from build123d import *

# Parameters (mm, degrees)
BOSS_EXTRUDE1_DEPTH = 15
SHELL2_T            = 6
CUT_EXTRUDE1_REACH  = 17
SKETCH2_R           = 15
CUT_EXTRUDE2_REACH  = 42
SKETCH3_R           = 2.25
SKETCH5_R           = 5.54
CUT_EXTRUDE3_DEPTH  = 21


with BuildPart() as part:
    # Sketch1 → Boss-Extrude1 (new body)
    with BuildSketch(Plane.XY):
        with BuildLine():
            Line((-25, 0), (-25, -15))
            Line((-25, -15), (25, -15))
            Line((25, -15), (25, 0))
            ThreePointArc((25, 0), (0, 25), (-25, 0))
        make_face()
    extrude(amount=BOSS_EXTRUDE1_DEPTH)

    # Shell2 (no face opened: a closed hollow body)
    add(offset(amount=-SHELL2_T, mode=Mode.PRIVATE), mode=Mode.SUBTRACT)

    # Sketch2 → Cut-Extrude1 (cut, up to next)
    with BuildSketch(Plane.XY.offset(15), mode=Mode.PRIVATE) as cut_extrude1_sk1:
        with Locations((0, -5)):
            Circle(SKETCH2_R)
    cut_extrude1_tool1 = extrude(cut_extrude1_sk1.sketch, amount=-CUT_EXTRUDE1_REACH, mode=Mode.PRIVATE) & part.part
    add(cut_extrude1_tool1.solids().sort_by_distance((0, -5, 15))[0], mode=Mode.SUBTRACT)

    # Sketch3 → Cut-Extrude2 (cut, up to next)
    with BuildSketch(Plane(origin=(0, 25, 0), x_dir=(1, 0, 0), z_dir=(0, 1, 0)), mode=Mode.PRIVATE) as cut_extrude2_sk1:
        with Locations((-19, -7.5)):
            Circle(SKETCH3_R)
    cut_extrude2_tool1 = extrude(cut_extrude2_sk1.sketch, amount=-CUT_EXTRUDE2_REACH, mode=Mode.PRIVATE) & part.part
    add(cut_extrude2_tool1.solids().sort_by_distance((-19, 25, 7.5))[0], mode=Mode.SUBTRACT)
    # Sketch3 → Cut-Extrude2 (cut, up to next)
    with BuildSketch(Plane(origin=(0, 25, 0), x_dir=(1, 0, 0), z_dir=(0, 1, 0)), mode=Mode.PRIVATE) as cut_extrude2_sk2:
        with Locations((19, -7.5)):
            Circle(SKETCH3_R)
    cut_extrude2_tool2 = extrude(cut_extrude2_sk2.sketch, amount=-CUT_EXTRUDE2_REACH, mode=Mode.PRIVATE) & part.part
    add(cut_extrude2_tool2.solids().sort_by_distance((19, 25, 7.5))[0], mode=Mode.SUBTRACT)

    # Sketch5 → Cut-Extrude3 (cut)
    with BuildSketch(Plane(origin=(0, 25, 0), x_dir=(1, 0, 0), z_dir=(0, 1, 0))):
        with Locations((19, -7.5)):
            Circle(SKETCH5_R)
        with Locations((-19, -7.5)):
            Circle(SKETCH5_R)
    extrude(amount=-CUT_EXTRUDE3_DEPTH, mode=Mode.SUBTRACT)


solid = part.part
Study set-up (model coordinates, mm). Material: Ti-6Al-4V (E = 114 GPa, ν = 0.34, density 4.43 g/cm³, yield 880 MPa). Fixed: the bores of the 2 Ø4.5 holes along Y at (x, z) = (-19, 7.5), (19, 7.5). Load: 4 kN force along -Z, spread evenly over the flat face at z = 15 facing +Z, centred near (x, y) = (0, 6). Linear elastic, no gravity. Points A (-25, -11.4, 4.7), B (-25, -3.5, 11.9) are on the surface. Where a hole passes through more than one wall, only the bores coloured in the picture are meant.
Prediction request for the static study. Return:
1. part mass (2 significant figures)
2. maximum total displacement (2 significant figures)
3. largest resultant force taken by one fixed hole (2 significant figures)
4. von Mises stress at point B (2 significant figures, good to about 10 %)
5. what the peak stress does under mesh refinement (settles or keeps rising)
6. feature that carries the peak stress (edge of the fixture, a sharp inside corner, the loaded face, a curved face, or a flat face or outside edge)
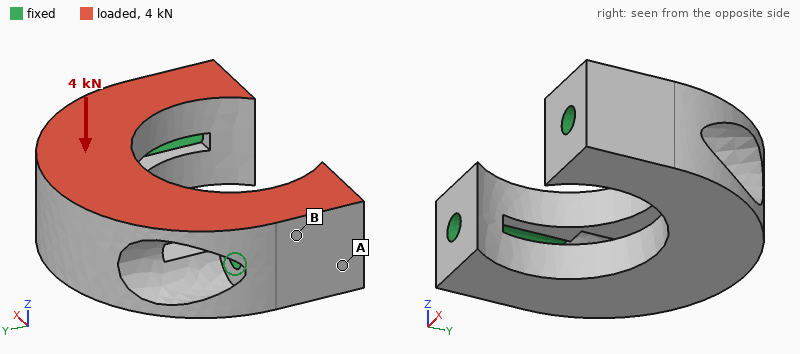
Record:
56 g
43 µm
2.0 kN
22 MPa
keeps rising
edge of the fixture
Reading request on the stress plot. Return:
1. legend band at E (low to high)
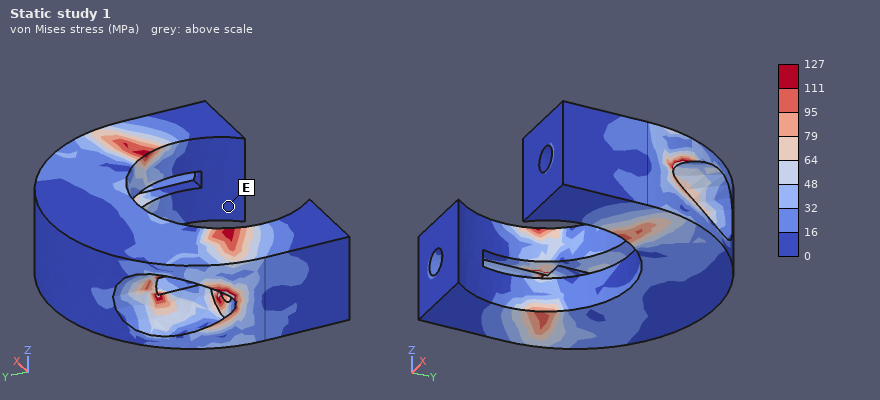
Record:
0 to 16 MPa
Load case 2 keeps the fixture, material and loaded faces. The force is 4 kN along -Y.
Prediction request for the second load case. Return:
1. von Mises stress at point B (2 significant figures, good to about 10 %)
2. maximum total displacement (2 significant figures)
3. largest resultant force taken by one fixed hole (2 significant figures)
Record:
19 MPa
21 µm
2.1 kN
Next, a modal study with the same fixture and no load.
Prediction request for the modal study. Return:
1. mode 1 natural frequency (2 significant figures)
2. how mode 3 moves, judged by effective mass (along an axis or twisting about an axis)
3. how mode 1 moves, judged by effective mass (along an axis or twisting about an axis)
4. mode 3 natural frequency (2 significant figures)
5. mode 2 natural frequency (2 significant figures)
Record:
7300 Hz
along X
along Z
18 kHz
17 kHz
